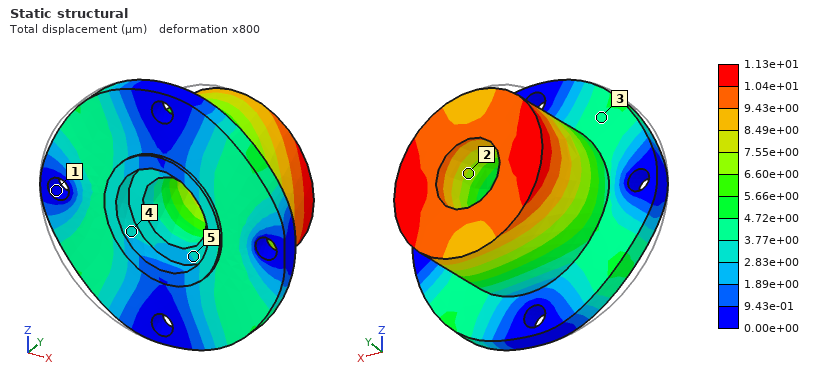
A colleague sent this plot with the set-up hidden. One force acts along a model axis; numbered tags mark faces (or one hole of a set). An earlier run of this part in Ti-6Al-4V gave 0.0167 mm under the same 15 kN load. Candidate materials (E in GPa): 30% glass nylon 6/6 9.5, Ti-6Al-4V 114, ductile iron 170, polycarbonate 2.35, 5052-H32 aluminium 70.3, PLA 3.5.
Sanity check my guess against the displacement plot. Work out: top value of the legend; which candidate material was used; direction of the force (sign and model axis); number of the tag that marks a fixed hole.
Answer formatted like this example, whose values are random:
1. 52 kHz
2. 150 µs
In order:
1. 1.13e+01 µm
2. ductile iron
3. +X
4. 1
